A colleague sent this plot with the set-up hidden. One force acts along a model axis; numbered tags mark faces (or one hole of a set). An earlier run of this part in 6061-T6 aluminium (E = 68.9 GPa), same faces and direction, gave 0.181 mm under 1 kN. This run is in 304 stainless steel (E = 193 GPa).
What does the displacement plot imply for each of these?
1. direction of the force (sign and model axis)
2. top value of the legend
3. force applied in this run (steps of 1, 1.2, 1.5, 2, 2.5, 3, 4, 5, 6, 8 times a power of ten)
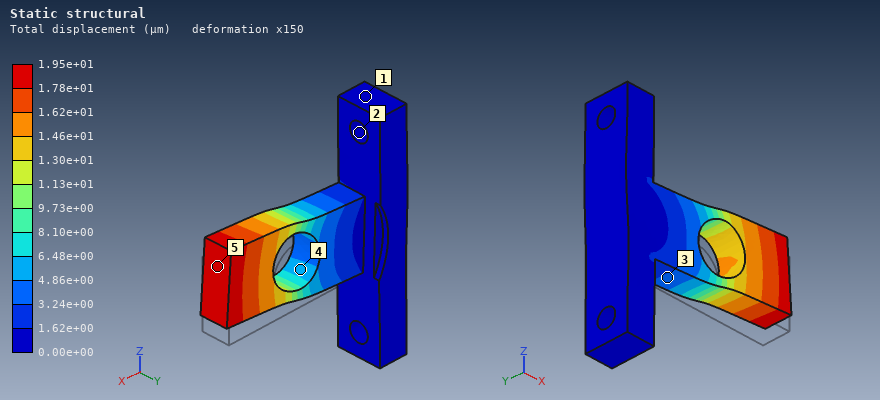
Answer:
+Z
1.95e+01 µm
300 N
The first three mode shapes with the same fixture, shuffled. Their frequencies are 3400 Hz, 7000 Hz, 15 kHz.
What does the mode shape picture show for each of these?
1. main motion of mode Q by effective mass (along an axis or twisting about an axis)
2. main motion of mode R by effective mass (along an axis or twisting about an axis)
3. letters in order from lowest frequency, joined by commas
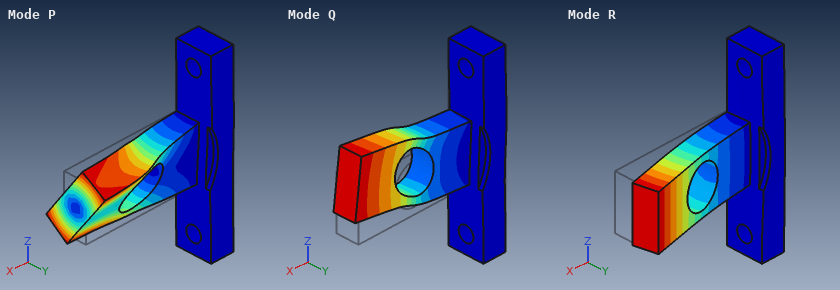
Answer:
along Z
along Y
R, Q, P
